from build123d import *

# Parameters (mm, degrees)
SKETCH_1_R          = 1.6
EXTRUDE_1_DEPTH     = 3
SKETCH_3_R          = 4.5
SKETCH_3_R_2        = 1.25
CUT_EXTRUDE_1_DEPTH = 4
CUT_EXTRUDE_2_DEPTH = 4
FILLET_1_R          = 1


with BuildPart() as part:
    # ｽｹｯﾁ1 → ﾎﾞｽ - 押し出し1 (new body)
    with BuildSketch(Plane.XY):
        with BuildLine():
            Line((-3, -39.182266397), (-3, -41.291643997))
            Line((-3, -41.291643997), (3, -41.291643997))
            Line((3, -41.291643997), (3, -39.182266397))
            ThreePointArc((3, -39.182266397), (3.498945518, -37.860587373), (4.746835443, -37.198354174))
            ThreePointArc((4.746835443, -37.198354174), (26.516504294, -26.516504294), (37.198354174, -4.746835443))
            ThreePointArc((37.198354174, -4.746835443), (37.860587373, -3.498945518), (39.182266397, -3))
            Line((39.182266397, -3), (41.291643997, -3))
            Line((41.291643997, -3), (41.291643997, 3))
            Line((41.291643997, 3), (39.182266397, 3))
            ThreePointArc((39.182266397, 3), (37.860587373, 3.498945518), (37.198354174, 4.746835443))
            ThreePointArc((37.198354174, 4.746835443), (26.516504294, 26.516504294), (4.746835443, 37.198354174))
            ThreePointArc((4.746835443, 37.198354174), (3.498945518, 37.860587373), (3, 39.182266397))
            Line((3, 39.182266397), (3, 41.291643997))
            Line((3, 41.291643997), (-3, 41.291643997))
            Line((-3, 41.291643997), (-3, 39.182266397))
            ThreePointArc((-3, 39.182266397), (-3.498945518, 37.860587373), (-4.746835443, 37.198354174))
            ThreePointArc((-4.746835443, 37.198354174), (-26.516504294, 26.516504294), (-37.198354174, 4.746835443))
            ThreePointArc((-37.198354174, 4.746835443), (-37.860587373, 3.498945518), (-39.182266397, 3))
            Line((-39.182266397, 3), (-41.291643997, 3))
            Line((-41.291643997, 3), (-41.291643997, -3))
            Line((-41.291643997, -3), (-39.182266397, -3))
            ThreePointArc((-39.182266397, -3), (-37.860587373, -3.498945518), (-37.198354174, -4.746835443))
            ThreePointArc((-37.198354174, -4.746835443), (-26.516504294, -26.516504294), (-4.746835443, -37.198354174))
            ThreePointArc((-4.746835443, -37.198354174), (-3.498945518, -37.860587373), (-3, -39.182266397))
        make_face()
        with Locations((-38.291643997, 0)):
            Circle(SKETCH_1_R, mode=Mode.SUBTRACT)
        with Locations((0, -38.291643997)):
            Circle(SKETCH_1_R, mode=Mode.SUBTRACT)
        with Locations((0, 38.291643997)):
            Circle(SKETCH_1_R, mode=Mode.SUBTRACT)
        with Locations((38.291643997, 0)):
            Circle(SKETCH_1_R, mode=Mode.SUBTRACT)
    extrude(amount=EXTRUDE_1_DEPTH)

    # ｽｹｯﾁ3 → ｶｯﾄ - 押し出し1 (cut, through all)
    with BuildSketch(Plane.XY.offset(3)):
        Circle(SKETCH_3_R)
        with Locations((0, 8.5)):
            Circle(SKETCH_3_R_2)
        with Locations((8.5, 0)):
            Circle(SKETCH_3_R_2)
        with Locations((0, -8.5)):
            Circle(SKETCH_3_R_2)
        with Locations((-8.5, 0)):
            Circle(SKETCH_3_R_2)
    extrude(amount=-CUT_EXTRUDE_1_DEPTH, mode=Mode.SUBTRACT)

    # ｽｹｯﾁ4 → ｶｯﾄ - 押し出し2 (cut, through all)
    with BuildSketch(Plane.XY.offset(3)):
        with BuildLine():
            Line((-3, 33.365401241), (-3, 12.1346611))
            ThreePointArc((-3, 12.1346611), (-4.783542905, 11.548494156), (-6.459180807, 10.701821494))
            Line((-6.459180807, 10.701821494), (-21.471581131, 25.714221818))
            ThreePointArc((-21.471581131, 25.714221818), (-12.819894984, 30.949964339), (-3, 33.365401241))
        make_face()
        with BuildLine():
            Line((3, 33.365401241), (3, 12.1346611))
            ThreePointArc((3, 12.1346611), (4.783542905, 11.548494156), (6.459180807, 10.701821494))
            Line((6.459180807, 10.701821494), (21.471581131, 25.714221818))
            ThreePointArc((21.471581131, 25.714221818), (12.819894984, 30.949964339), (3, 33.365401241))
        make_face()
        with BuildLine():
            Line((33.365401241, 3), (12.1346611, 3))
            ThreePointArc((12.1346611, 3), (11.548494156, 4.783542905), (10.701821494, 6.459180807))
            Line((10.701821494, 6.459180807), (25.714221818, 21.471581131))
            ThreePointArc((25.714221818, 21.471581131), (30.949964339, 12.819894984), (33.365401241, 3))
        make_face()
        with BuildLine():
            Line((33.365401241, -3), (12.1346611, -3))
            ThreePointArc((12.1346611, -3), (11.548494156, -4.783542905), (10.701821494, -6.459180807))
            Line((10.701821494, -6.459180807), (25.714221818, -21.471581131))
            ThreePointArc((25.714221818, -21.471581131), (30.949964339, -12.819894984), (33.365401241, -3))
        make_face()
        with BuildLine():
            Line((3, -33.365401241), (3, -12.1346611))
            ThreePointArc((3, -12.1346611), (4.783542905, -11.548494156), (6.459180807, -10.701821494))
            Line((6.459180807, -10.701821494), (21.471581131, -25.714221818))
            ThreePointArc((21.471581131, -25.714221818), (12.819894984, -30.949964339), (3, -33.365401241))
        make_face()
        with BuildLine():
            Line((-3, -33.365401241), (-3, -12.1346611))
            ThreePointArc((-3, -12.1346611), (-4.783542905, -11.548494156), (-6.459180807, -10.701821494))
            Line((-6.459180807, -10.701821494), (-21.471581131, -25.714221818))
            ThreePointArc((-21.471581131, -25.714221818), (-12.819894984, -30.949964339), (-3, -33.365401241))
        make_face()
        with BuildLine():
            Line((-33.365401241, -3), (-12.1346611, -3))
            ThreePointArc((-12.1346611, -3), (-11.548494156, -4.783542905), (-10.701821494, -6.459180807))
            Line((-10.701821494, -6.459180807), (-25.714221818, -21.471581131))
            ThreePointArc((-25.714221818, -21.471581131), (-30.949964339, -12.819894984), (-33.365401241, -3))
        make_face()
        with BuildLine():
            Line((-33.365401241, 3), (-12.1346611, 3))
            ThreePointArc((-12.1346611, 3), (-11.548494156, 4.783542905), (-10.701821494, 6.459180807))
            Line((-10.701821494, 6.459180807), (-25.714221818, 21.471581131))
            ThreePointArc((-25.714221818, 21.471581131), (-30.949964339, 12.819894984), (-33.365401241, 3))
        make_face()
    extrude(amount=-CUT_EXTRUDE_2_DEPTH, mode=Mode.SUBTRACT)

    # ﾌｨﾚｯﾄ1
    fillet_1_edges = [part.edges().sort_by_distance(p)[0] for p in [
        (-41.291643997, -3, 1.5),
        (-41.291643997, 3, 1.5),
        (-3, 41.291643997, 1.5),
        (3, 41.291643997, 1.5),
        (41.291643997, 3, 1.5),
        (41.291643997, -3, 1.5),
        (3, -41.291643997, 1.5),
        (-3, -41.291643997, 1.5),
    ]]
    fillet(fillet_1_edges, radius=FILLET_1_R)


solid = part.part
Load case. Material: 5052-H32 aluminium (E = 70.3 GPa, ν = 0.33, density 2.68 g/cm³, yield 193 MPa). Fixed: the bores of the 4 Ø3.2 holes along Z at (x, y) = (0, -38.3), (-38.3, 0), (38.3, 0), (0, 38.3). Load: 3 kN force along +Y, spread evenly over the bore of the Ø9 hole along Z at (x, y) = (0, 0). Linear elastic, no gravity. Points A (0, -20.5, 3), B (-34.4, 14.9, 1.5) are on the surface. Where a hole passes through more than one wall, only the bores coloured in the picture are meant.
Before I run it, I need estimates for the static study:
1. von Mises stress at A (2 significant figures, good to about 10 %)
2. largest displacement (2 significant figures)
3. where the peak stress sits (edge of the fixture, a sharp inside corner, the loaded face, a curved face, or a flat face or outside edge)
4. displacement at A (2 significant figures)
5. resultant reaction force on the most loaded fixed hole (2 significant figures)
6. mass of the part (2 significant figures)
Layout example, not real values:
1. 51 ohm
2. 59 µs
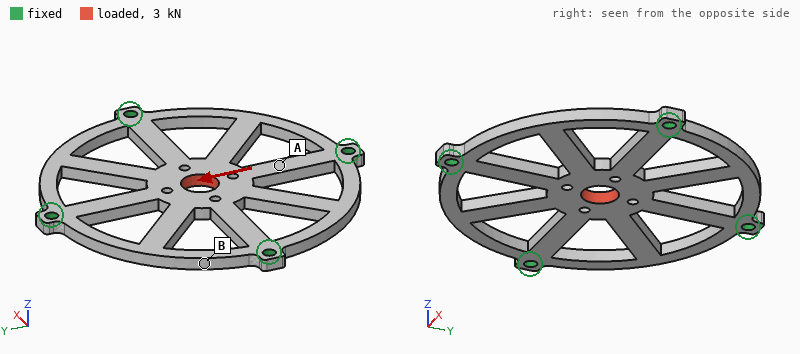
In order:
1. 67 MPa
2. 32 µm
3. a curved face
4. 16 µm
5. 1.1 kN
6. 19 g
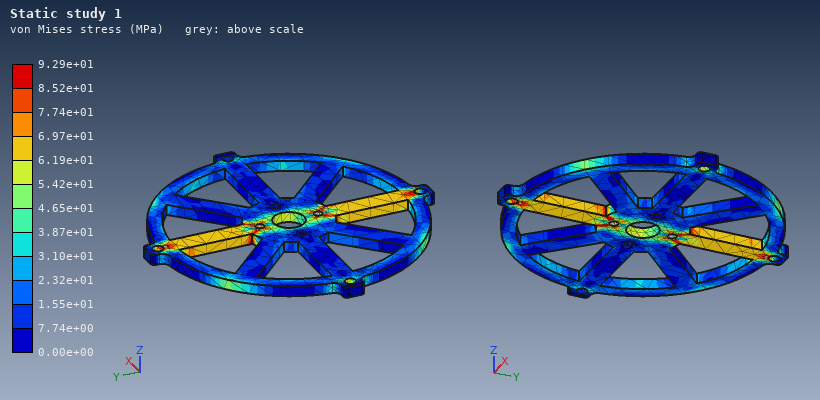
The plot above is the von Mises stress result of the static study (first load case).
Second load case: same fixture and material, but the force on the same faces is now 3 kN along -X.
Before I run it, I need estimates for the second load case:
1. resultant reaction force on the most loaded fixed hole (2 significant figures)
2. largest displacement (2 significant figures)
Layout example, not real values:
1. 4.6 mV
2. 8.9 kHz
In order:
1. 1.1 kN
2. 32 µm
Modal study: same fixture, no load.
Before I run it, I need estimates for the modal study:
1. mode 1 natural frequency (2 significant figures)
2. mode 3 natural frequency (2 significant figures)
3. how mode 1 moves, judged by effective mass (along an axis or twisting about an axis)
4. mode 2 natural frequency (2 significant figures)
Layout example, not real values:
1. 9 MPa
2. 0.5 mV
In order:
1. 2900 Hz
2. 4400 Hz
3. along Z
4. 4400 Hz
